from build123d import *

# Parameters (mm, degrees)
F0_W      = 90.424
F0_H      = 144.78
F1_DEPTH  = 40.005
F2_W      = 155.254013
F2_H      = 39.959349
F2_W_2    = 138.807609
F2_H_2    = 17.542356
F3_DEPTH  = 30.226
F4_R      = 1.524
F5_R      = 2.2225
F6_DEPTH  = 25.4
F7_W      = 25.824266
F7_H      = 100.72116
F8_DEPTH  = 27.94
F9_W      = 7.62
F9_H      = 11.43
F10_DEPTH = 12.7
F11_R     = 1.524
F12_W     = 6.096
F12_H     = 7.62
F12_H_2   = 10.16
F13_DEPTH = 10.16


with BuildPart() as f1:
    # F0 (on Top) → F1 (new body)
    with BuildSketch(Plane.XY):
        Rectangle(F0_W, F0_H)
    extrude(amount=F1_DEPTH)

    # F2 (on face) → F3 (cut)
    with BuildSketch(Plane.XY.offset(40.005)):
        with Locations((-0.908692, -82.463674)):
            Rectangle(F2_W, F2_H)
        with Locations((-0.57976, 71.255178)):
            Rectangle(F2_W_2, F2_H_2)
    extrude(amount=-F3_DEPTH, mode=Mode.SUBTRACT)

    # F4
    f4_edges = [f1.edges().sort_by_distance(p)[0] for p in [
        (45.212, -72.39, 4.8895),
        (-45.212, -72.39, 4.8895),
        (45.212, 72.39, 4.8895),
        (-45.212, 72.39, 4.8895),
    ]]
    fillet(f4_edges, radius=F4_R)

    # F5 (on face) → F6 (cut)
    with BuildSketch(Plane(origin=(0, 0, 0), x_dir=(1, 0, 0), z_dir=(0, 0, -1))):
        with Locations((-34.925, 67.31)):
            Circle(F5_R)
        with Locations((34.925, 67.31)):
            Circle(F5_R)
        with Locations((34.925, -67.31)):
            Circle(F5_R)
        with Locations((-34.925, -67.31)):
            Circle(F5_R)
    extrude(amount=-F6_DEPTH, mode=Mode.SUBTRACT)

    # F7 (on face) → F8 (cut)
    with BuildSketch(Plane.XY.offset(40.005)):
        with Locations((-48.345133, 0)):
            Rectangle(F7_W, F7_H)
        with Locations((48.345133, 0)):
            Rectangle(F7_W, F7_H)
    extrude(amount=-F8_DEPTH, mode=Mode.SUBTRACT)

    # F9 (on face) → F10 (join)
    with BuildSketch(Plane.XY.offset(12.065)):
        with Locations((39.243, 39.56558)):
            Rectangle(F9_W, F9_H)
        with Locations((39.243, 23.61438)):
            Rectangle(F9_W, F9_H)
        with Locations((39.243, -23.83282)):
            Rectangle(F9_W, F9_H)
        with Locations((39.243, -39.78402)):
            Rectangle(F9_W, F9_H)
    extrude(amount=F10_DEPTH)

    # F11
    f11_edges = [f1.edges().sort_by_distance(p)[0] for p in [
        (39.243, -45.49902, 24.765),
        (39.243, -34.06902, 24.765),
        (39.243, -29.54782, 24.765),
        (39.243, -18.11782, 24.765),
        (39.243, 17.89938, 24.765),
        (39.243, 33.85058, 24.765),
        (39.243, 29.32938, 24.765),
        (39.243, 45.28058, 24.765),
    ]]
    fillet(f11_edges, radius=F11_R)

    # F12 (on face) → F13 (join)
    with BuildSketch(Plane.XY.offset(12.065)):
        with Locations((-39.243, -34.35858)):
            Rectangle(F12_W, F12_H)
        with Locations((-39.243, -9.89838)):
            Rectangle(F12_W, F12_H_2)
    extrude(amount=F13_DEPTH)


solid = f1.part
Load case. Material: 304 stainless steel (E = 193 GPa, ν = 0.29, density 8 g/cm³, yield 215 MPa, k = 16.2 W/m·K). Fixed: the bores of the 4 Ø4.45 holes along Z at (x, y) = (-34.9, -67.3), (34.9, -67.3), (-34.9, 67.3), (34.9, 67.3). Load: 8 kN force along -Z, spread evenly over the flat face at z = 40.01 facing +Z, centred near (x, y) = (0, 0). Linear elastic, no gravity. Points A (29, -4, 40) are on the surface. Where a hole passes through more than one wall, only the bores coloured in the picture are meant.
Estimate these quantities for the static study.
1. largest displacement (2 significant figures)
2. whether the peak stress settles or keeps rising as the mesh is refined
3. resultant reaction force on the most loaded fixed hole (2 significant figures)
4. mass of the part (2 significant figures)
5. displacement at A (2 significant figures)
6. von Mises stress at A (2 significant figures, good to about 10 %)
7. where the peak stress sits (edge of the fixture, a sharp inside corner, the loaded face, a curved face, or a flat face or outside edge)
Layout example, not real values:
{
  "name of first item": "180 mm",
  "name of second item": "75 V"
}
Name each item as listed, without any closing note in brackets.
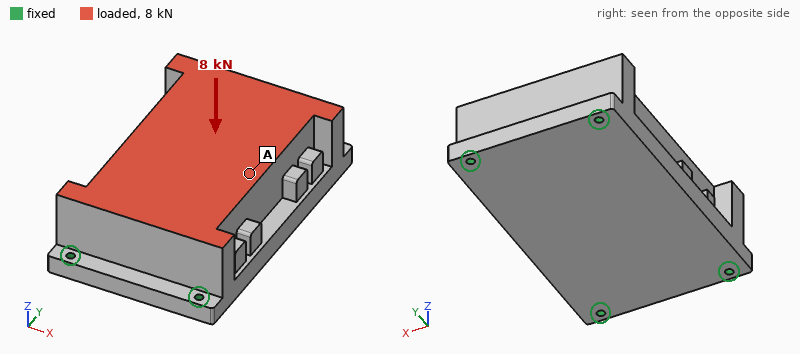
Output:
{
  "largest displacement": "4.8 µm",
  "whether the peak stress settles or keeps rising as the mesh is refined": "keeps rising",
  "resultant reaction force on the most loaded fixed hole": "2.4 kN",
  "mass of the part": "3.4 kg",
  "displacement at A": "4.6 µm",
  "von Mises stress at A": "5.0 MPa",
  "where the peak stress sits": "edge of the fixture"
}
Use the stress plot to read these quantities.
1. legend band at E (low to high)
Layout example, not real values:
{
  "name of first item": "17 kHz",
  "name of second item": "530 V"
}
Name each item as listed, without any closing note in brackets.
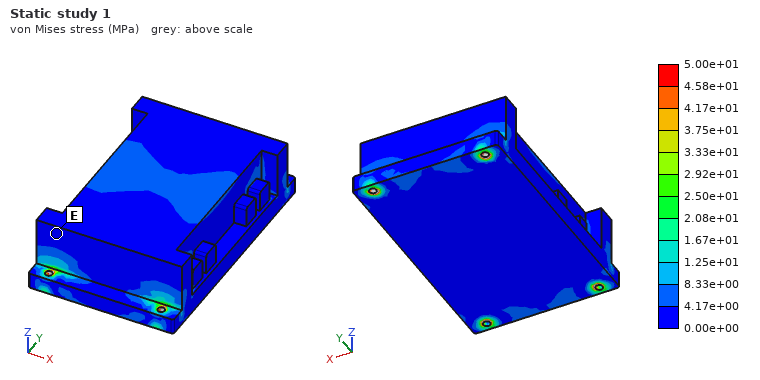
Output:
{
  "legend band at E": "0.00e+00 to 4.17e+00 MPa"
}
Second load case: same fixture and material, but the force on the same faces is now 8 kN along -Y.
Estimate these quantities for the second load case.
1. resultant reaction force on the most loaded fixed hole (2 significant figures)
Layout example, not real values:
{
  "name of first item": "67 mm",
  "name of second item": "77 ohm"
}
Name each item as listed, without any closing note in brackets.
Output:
{
  "resultant reaction force on the most loaded fixed hole": "2.4 kN"
}
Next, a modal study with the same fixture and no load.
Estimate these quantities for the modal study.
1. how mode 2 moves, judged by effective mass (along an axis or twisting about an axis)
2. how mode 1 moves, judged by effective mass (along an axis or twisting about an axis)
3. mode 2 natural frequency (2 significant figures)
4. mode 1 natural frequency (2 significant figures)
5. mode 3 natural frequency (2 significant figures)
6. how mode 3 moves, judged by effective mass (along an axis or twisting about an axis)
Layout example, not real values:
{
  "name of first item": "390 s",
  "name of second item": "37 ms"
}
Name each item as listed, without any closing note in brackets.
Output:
{
  "how mode 2 moves, judged by effective mass": "along X",
  "how mode 1 moves, judged by effective mass": "along Z",
  "mode 2 natural frequency": "4800 Hz",
  "mode 1 natural frequency": "3900 Hz",
  "mode 3 natural frequency": "6400 Hz",
  "how mode 3 moves, judged by effective mass": "along X"
}
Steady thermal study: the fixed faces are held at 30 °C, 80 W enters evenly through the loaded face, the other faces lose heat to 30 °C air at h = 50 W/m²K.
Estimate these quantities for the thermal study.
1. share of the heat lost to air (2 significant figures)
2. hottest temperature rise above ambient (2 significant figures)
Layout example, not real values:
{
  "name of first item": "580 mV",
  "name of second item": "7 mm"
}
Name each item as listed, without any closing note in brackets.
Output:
{
  "share of the heat lost to air": "65 %",
  "hottest temperature rise above ambient": "49 K"
}
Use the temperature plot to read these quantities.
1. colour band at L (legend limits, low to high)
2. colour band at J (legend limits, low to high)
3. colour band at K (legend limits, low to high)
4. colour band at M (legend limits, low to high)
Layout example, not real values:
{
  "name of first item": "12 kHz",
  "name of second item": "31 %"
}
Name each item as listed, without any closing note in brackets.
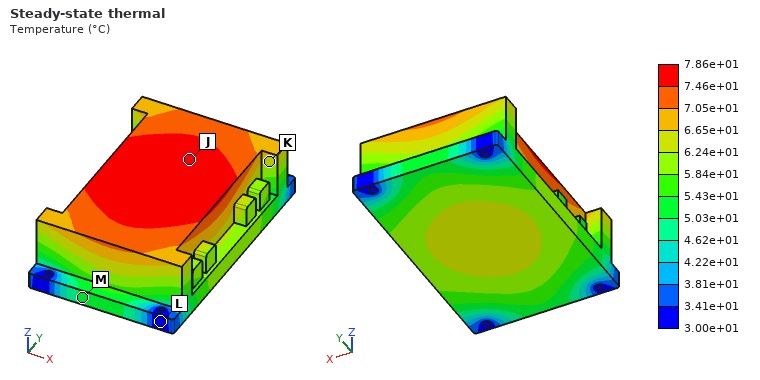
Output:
{
  "colour band at L": "3.00e+01 to 3.41e+01 °C",
  "colour band at J": "7.46e+01 to 7.86e+01 °C",
  "colour band at K": "6.24e+01 to 6.65e+01 °C",
  "colour band at M": "5.03e+01 to 5.43e+01 °C"
}
